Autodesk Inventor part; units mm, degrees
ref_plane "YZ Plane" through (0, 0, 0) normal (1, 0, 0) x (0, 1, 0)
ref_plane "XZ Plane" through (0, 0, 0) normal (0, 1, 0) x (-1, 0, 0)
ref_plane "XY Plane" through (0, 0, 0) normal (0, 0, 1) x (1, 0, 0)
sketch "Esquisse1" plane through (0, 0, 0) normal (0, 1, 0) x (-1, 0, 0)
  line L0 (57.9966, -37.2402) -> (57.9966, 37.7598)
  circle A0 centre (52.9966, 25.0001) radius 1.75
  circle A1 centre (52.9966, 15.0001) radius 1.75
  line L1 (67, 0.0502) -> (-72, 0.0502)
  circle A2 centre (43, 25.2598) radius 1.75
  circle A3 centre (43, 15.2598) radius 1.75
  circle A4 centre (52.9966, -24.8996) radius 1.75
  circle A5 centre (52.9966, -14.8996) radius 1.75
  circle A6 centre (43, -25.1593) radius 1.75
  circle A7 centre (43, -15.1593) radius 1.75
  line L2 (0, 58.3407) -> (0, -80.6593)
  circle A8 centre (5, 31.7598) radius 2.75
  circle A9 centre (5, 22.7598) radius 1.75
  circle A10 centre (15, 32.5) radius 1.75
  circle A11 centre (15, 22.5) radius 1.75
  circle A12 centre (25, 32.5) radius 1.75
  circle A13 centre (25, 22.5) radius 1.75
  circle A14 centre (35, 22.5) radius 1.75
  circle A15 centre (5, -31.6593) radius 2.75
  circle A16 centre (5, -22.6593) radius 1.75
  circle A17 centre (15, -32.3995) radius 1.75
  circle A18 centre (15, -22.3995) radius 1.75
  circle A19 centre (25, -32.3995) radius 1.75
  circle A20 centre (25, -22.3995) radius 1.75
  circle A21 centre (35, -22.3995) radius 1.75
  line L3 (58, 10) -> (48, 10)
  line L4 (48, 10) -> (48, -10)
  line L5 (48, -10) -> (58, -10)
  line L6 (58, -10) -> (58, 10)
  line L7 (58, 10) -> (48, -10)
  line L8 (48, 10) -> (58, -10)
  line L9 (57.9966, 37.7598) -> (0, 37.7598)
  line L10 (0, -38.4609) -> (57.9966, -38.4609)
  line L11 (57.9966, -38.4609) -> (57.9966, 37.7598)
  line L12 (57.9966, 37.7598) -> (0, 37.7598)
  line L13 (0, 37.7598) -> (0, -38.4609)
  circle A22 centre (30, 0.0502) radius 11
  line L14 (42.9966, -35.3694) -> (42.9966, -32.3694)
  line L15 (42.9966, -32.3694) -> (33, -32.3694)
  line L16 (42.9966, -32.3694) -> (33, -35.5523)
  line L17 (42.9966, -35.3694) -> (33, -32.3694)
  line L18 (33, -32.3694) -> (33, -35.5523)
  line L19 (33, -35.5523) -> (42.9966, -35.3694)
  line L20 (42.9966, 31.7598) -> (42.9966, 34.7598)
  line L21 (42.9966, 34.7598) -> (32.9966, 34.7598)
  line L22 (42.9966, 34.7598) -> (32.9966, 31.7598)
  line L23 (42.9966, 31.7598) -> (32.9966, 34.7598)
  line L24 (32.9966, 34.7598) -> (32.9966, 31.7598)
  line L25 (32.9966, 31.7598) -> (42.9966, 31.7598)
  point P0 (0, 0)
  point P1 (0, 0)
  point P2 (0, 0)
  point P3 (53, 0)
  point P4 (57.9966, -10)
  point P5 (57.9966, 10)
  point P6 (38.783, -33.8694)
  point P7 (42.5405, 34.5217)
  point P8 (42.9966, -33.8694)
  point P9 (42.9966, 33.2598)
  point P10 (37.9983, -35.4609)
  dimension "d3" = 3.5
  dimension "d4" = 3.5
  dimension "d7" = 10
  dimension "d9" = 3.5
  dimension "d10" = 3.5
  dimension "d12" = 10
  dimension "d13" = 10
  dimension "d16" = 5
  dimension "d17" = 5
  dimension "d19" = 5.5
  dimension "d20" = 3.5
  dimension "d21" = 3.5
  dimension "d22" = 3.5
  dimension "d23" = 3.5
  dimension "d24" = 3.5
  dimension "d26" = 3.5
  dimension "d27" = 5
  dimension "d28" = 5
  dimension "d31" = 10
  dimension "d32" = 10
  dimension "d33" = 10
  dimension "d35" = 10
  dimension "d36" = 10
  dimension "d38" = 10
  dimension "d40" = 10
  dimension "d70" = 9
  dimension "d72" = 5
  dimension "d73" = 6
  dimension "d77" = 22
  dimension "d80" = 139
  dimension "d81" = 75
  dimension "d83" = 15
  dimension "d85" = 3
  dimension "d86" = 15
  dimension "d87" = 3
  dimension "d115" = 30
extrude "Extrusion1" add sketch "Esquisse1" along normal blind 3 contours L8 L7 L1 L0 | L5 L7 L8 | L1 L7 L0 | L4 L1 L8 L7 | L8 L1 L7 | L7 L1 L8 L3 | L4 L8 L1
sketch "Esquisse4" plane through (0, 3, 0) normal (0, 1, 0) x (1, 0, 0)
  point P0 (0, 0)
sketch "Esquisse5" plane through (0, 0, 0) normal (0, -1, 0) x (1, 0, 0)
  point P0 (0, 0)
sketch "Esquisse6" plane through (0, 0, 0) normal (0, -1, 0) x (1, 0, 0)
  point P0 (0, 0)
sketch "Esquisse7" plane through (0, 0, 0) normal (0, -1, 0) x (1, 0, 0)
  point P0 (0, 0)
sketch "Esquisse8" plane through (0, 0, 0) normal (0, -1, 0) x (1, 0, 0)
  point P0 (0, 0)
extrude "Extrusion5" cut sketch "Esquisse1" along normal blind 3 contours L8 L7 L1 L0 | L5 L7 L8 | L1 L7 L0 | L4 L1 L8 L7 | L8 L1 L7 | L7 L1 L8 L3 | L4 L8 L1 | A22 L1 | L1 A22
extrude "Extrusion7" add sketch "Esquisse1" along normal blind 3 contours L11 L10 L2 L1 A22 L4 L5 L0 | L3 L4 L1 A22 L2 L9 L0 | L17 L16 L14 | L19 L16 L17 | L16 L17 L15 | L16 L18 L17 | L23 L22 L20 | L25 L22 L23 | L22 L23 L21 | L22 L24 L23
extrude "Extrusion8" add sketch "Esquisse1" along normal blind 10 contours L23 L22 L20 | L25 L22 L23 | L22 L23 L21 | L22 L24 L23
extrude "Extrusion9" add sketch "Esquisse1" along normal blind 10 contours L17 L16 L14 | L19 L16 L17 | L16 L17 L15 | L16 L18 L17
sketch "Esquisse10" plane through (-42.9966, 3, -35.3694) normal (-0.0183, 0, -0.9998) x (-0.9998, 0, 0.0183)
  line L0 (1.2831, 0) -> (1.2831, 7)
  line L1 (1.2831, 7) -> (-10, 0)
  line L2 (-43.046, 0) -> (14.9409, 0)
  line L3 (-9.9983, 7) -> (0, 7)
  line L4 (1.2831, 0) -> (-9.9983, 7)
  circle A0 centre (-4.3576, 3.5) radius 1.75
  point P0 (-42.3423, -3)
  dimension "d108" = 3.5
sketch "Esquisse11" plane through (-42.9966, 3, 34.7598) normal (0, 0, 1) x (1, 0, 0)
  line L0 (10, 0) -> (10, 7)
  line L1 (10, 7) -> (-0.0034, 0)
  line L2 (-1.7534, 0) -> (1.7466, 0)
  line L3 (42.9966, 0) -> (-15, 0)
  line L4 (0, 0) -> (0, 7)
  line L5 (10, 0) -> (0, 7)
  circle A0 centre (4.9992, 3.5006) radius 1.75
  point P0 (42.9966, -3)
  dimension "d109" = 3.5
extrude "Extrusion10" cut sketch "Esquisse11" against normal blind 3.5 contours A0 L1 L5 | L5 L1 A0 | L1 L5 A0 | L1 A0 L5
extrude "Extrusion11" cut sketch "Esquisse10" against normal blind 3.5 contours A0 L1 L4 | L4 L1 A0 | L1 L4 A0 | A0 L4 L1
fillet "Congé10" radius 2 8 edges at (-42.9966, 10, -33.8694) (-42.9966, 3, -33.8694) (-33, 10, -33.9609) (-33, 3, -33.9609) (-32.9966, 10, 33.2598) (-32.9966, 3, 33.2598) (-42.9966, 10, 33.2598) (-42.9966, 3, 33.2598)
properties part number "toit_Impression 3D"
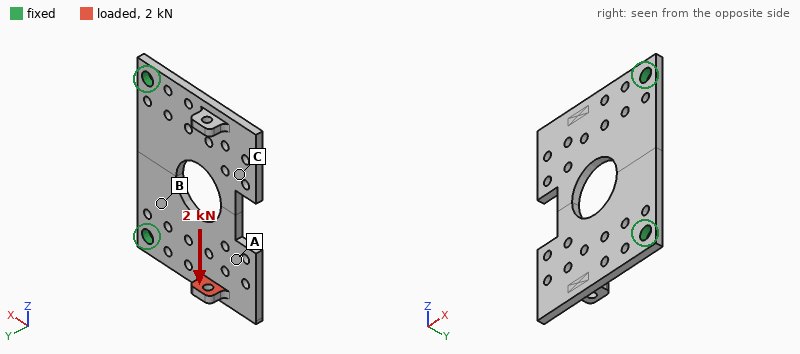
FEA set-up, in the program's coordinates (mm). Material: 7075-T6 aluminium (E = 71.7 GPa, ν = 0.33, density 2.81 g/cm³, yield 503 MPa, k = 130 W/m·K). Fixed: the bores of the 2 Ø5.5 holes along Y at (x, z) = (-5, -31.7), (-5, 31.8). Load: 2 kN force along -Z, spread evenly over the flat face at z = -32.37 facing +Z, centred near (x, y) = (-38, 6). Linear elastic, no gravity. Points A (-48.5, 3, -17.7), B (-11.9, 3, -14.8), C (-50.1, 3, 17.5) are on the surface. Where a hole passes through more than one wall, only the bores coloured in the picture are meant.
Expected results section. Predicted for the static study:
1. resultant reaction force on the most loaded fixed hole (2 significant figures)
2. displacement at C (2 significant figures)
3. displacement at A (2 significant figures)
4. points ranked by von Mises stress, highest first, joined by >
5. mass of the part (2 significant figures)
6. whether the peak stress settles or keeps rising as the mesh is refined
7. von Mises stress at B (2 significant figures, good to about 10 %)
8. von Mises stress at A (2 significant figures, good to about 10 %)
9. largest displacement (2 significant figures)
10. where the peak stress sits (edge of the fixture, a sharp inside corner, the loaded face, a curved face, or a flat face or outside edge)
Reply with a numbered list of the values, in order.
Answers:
1. 1.4 kN
2. 0.39 mm
3. 0.18 mm
4. A > B > C
5. 31 g
6. keeps rising
7. 52 MPa
8. 130 MPa
9. 0.62 mm
10. a sharp inside corner
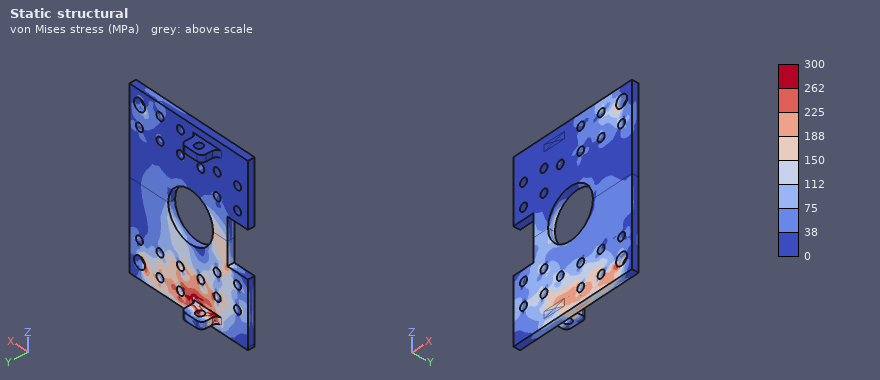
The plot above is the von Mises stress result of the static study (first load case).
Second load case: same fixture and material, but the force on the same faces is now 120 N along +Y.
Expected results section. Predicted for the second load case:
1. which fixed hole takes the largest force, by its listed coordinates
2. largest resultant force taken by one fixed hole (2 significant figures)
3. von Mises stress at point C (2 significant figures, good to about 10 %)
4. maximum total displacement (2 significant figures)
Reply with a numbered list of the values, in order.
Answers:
1. (-5, -31.7)
2. 120 N
3. 7.6 MPa
4. 0.55 mm
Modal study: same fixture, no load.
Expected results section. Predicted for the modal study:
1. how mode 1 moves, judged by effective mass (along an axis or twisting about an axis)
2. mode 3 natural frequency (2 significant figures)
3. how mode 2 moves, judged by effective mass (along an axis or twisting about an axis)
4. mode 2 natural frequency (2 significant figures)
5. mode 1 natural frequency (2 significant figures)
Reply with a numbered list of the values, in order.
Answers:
1. along Y
2. 2900 Hz
3. twisting about X
4. 1400 Hz
5. 760 Hz
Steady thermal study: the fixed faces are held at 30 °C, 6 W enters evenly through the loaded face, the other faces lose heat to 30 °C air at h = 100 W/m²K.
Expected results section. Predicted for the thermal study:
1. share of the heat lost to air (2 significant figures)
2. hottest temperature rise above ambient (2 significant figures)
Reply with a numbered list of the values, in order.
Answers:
1. 56 %
2. 21 K
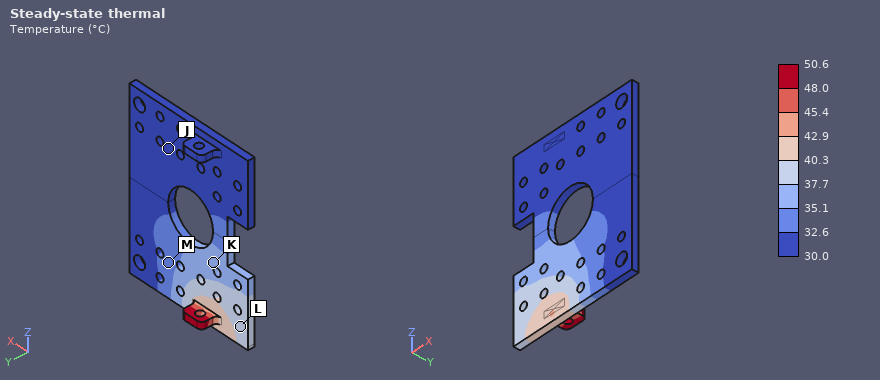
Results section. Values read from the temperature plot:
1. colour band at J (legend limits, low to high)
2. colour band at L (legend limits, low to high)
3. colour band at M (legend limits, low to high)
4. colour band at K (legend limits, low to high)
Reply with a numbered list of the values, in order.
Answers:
1. 30.0 to 32.6 °C
2. 37.7 to 40.3 °C
3. 32.6 to 35.1 °C
4. 35.1 to 37.7 °C
